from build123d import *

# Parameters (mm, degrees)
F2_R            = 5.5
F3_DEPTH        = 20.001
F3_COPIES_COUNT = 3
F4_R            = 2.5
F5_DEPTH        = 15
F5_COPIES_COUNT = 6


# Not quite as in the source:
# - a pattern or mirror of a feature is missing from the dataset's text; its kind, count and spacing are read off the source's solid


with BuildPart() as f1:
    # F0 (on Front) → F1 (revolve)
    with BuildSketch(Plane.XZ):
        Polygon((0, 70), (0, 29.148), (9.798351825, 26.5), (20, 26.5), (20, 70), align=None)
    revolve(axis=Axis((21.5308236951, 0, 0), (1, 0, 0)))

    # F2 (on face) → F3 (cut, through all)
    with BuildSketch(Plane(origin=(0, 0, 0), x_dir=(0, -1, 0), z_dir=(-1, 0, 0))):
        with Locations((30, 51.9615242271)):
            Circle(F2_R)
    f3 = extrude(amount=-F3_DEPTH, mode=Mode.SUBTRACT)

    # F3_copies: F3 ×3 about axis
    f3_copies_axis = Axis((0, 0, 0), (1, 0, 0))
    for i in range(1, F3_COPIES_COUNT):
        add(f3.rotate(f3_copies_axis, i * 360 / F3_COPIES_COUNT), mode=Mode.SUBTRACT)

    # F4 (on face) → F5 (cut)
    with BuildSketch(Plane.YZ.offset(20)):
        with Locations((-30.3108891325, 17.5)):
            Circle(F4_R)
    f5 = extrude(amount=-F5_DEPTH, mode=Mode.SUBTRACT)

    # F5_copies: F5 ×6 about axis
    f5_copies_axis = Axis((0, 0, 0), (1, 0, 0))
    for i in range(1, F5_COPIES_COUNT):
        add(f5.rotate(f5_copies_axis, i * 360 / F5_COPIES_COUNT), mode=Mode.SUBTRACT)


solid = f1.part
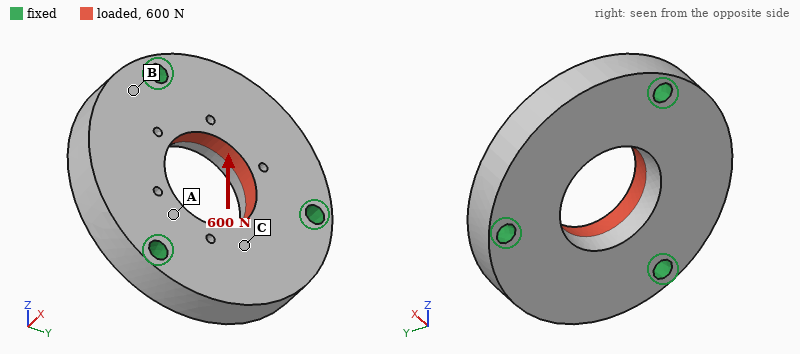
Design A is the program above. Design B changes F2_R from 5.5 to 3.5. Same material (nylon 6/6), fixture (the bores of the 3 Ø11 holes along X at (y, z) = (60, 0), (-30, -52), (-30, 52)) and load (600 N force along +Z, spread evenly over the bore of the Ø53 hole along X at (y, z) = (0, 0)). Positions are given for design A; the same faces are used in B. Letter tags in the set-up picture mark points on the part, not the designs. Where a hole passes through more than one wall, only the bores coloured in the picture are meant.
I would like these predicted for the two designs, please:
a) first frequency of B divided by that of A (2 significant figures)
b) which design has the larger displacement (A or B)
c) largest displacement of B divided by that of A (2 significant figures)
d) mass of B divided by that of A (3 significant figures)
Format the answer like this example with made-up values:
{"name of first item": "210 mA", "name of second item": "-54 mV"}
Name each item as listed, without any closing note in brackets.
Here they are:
{"first frequency of B divided by that of A": "0.89", "which design has the larger displacement": "B", "largest displacement of B divided by that of A": "1.1", "mass of B divided by that of A": "1.01"}
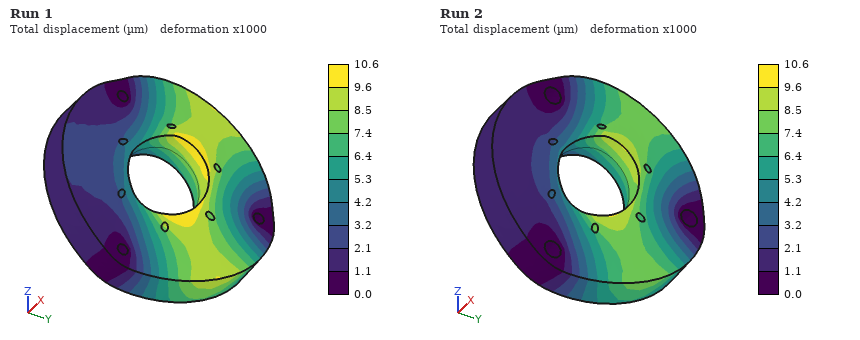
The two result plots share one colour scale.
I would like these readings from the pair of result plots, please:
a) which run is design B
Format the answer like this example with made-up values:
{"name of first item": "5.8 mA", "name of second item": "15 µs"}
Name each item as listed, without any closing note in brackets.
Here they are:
{"which run is design B": "Run 1"}
